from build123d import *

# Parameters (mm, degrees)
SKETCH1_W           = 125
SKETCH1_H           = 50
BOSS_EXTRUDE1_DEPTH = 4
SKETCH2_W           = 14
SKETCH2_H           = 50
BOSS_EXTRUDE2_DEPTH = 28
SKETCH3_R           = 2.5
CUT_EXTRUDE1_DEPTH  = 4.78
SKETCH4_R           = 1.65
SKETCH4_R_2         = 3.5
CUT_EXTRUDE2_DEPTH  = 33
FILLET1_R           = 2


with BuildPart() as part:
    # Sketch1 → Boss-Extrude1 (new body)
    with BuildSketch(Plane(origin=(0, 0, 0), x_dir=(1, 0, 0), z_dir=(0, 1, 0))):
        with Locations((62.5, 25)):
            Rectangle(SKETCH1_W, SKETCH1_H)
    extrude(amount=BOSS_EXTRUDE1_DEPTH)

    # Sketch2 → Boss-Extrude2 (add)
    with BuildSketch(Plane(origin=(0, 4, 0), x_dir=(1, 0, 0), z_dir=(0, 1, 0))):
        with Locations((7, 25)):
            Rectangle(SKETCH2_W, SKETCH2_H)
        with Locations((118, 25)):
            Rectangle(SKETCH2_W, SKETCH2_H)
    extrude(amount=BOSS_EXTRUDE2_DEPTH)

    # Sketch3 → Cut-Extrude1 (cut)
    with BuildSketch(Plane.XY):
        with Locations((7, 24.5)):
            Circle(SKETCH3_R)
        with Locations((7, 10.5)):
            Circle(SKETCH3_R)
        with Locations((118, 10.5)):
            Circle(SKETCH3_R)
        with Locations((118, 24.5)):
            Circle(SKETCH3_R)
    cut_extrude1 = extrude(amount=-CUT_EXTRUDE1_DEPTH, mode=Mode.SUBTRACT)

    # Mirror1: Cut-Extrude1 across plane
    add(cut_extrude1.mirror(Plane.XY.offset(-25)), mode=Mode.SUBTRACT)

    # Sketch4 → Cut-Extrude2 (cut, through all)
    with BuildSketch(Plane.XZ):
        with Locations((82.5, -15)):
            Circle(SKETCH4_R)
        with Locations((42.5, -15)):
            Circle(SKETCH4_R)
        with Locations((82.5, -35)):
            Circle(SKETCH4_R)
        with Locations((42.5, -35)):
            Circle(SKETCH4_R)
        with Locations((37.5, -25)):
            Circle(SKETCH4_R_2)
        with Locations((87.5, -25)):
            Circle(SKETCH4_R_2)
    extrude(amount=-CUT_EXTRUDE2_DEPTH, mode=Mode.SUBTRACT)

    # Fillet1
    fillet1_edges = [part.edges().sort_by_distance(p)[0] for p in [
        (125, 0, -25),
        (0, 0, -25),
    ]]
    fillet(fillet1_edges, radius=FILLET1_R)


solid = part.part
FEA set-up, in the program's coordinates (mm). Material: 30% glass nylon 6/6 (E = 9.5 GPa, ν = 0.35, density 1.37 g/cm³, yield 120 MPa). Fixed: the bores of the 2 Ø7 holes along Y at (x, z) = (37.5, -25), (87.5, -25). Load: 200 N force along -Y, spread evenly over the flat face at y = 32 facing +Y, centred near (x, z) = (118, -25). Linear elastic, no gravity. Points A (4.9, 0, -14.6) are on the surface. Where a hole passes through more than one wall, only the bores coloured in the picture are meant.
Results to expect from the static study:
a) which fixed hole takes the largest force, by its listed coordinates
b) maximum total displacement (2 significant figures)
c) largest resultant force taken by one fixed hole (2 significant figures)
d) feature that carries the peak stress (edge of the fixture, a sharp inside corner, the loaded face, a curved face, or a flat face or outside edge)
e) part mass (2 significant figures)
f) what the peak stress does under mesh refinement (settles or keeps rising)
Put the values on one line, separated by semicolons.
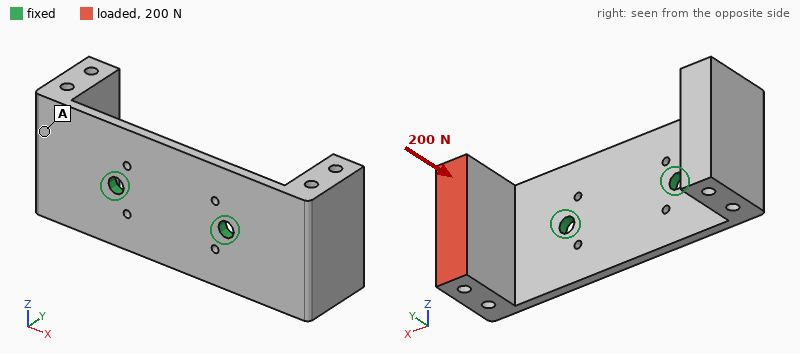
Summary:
(87.5, -25); 1.5 mm; 230 N; edge of the fixture; 86 g; keeps rising
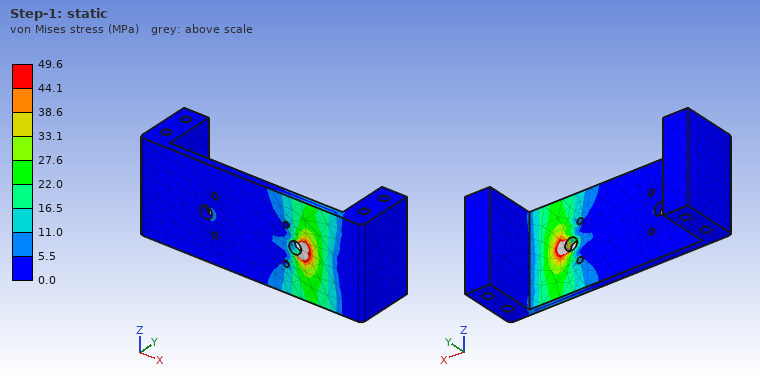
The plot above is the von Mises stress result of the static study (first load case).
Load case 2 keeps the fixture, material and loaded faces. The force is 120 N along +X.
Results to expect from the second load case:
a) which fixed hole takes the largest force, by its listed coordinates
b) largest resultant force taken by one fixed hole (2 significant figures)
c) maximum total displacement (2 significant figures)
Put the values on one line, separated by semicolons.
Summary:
(87.5, -25); 99 N; 1.4 mm
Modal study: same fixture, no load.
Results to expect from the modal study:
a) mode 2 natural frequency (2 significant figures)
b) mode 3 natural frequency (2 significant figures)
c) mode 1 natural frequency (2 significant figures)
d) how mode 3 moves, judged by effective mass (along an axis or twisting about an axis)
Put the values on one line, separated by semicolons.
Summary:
360 Hz; 600 Hz; 360 Hz; along Z
